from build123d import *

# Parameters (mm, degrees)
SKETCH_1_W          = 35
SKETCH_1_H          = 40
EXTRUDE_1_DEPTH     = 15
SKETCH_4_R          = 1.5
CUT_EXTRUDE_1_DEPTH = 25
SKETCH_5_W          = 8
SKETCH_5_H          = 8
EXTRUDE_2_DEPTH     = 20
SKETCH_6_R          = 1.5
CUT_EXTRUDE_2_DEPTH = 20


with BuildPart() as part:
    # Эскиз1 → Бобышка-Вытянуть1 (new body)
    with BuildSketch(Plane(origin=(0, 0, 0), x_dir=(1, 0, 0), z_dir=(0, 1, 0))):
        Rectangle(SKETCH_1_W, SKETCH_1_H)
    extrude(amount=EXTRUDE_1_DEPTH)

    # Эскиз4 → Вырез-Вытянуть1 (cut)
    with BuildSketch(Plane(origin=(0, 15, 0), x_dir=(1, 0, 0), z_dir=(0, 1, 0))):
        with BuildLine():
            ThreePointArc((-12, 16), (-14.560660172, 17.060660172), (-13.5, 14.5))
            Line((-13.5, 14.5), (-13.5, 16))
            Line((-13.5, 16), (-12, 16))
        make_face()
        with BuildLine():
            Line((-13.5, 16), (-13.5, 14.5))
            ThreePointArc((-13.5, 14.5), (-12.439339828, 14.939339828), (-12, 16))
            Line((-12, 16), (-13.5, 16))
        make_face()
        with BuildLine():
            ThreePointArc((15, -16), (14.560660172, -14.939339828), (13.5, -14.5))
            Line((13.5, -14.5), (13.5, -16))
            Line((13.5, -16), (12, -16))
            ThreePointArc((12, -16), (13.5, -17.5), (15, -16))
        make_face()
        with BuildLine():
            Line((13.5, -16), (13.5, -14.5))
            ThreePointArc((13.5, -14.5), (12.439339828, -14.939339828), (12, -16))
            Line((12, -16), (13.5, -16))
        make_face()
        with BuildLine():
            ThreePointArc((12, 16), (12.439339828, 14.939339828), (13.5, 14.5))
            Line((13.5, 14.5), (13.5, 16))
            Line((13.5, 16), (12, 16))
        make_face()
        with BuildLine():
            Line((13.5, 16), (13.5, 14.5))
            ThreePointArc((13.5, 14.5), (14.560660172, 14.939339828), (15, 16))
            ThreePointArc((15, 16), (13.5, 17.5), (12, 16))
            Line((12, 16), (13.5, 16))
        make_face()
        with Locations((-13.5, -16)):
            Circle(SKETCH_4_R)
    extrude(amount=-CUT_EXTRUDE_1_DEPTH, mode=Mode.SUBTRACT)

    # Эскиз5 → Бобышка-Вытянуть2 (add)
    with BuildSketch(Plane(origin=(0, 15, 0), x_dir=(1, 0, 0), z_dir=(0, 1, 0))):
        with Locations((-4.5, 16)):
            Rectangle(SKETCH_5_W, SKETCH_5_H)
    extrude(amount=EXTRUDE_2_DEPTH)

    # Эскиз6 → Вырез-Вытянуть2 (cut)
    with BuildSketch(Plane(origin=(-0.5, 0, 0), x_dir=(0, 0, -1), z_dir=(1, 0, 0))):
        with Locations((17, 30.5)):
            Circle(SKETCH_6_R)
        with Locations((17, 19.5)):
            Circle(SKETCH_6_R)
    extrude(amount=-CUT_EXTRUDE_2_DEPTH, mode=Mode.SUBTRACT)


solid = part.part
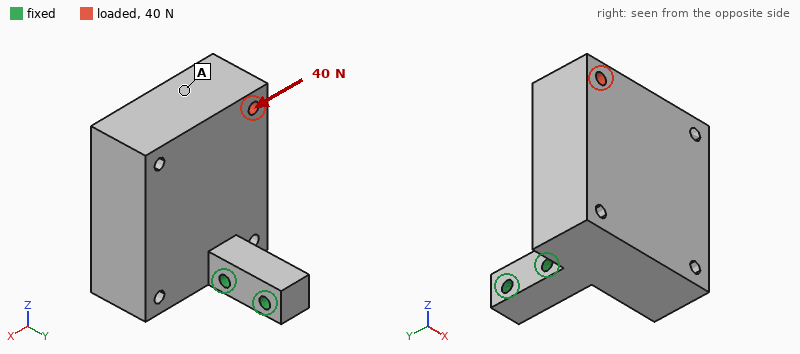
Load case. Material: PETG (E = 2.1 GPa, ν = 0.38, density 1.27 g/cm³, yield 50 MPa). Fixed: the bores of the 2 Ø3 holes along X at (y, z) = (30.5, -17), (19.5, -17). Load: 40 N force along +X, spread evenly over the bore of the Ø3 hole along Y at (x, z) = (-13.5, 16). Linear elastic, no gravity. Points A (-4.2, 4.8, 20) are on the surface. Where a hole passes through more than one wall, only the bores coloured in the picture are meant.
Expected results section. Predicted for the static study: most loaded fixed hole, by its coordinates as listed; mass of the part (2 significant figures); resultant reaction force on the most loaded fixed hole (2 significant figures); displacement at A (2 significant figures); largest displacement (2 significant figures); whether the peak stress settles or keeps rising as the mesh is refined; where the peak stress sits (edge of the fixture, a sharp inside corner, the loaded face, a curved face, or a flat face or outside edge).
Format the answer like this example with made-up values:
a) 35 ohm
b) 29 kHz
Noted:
a) (19.5, -17)
b) 28 g
c) 42 N
d) 0.61 mm
e) 0.72 mm
f) keeps rising
g) edge of the fixture
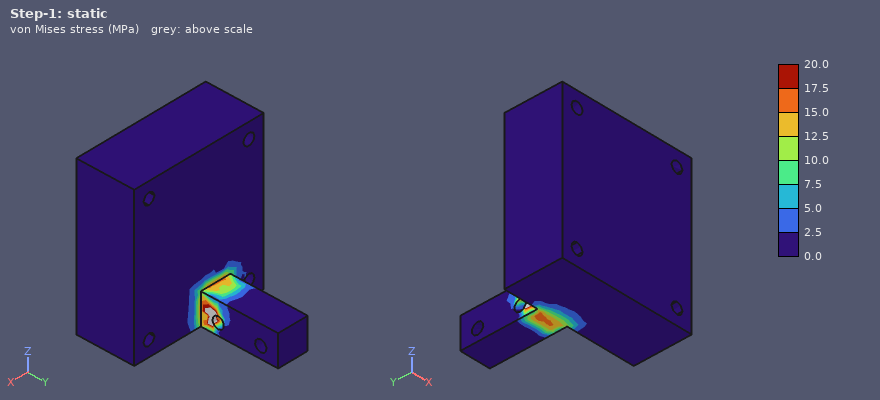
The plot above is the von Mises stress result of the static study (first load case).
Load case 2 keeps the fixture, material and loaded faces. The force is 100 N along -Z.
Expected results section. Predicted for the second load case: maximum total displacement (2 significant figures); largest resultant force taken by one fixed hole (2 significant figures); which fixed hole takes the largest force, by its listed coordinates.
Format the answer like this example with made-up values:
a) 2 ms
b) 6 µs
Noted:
a) 0.68 mm
b) 150 N
c) (19.5, -17)
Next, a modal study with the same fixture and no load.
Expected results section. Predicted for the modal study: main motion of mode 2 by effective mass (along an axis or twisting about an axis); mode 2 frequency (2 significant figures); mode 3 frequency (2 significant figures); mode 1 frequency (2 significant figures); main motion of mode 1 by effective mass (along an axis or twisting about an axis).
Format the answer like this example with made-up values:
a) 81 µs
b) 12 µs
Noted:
a) along Y
b) 400 Hz
c) 820 Hz
d) 370 Hz
e) along X
